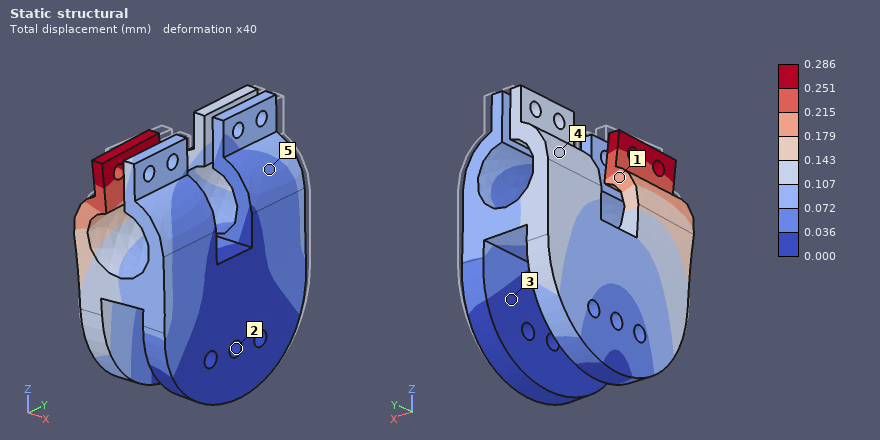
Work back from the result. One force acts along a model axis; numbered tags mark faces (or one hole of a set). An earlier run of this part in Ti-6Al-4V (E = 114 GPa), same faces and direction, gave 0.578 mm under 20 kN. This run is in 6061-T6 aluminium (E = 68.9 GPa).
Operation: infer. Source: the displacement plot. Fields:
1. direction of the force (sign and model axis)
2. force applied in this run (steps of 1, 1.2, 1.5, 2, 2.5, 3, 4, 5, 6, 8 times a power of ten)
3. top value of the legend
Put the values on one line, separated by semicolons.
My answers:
-Y; 6 kN; 0.286 mm
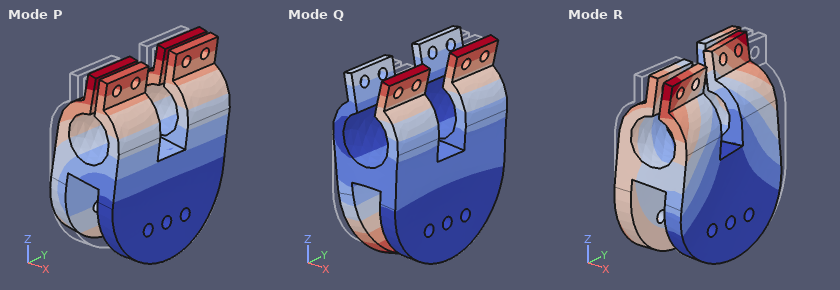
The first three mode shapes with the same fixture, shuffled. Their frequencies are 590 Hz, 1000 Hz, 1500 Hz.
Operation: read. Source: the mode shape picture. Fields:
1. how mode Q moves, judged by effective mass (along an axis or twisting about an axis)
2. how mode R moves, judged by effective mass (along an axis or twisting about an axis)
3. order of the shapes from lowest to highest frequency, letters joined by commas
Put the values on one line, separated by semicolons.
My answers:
along X; along Y; P, R, Q
